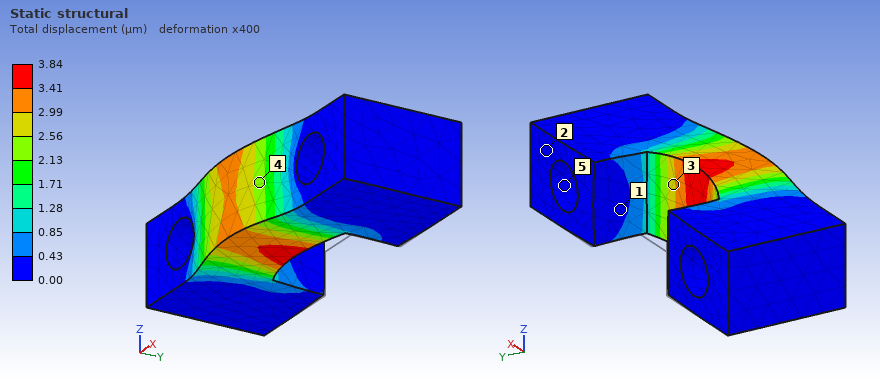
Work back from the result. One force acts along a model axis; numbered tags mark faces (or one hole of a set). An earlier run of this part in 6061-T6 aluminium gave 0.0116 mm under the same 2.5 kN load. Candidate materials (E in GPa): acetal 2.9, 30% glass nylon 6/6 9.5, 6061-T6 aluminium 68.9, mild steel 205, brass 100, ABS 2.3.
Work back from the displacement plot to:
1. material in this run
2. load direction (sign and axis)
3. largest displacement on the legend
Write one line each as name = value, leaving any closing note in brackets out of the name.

material in this run = mild steel
load direction = -Y
largest displacement on the legend = 3.84 µm
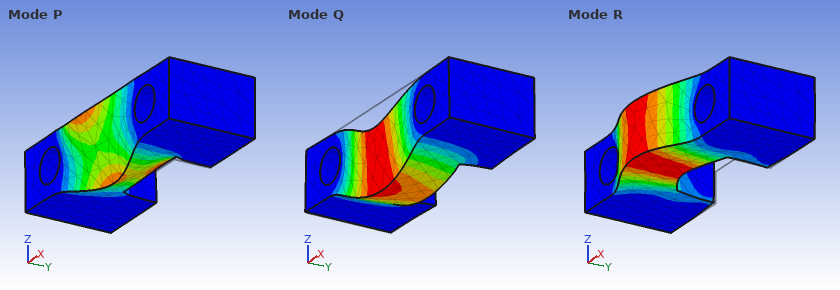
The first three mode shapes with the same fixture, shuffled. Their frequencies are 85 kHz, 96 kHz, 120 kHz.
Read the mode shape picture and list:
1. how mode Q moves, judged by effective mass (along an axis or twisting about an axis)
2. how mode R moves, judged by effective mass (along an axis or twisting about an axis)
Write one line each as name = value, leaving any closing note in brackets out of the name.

how mode Q moves, judged by effective mass = along Z
how mode R moves, judged by effective mass = along Y
